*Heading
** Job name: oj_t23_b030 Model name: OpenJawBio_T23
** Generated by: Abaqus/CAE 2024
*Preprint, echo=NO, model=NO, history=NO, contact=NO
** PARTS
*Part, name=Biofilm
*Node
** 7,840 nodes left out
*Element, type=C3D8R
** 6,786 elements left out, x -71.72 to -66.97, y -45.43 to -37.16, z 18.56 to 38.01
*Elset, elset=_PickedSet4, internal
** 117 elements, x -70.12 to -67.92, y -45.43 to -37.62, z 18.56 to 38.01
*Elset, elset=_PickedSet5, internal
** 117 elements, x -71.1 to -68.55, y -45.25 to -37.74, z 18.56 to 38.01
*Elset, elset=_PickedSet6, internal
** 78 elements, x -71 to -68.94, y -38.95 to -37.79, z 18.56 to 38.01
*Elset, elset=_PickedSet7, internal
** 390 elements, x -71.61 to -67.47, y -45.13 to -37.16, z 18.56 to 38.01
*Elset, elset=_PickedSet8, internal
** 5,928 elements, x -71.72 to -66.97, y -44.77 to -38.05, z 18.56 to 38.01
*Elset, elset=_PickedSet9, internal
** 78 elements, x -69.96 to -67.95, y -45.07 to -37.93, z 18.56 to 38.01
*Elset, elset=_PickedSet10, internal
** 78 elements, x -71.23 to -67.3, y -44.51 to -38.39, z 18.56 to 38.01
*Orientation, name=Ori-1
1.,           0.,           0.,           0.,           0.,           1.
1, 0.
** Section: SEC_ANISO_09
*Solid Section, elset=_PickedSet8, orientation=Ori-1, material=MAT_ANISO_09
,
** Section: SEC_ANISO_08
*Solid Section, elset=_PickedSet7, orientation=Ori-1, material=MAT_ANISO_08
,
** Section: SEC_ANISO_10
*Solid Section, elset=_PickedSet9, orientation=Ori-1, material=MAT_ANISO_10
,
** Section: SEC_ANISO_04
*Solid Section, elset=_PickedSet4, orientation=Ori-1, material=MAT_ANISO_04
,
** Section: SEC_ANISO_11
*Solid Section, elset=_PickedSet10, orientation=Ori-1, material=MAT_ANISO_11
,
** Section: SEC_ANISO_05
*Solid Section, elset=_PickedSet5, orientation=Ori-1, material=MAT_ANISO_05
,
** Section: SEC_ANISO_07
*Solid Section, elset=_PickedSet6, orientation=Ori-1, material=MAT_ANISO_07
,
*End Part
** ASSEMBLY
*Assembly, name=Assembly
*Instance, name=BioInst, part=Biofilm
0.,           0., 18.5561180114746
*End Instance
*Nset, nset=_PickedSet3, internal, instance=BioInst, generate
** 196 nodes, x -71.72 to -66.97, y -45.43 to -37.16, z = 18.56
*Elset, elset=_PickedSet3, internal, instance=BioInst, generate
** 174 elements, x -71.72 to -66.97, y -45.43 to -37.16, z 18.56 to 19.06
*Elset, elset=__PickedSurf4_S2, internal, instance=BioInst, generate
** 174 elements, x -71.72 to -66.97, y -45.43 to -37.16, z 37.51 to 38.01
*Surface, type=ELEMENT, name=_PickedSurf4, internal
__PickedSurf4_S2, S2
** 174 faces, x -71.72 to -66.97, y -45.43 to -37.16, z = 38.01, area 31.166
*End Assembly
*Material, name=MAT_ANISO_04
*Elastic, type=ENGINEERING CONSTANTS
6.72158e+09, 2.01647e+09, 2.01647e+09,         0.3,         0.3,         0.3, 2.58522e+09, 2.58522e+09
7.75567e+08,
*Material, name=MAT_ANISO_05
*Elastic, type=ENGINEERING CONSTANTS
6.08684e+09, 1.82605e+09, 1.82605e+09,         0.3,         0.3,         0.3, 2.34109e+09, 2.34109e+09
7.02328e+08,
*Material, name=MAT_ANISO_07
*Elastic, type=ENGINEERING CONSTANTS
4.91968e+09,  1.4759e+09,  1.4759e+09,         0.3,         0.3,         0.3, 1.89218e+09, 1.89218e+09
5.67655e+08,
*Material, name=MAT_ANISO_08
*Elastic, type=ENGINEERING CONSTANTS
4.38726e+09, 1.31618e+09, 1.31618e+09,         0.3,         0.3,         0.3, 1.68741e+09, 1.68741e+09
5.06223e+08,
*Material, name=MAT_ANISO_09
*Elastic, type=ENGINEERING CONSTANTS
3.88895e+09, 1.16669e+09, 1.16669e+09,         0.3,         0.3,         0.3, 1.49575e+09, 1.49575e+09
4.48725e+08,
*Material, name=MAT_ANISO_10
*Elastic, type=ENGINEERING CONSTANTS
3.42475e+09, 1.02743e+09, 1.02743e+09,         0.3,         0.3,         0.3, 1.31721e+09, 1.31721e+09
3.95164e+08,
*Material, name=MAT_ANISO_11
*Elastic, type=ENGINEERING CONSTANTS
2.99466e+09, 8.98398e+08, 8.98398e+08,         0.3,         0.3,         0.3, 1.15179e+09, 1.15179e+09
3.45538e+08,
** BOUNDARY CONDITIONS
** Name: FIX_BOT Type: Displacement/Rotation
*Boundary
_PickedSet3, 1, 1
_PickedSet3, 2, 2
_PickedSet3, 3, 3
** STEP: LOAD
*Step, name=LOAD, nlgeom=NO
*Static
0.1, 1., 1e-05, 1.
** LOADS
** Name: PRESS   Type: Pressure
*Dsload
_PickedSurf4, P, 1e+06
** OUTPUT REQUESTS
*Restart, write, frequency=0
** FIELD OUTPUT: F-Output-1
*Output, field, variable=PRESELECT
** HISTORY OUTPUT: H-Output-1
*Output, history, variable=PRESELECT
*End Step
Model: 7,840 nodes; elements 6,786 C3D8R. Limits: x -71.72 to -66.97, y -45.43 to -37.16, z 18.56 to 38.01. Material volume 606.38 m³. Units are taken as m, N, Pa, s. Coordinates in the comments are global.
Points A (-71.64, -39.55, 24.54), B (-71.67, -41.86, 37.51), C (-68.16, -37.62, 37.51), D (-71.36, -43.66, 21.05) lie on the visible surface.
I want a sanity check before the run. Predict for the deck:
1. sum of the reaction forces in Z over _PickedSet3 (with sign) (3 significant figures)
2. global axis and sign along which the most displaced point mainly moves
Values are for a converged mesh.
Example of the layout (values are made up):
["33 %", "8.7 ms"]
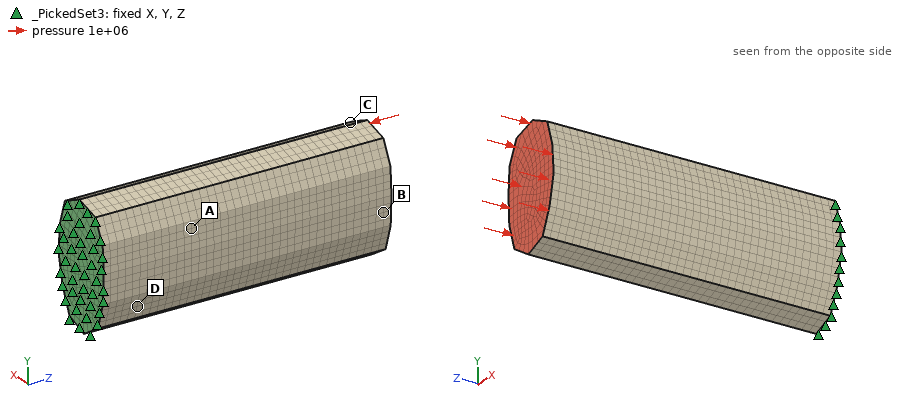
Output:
["3.12e+07 N", "-Z"]
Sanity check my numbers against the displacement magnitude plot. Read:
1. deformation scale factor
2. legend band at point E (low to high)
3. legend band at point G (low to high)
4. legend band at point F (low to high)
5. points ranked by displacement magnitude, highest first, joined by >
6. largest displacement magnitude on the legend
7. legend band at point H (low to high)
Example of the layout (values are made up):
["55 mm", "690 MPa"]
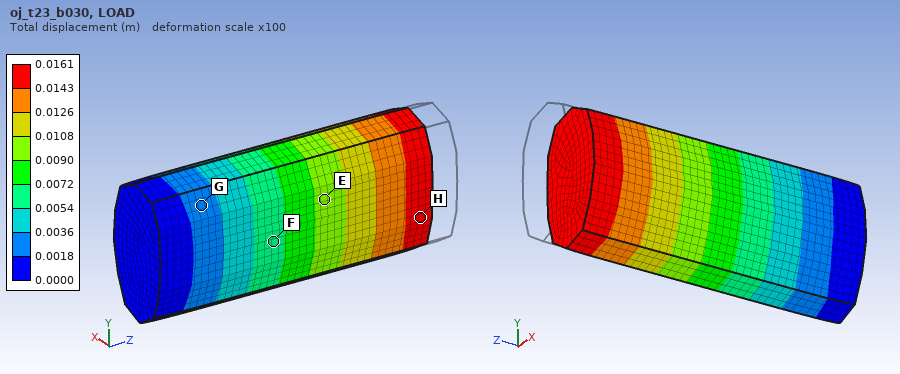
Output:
["100", "0.0090 to 0.0108 m", "0.0018 to 0.0036 m", "0.0054 to 0.0072 m", "H > E > F > G", "0.0161 m", "0.0143 to 0.0161 m"]
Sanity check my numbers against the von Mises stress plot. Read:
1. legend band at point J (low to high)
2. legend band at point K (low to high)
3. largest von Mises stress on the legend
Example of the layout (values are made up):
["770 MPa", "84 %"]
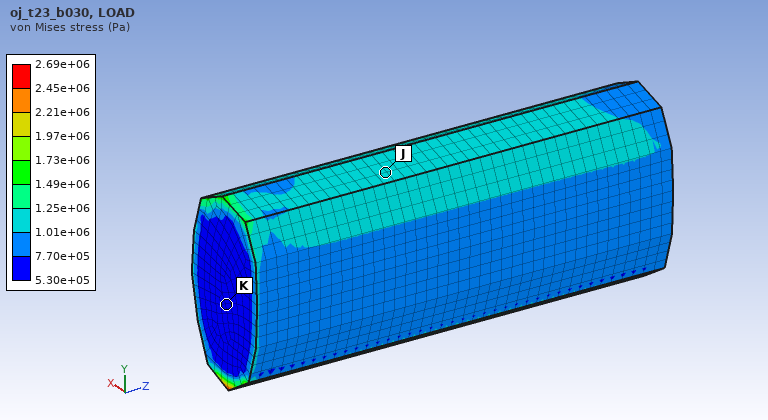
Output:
["1.01e+06 to 1.25e+06 Pa", "5.30e+05 to 7.70e+05 Pa", "2.69e+06 Pa"]
